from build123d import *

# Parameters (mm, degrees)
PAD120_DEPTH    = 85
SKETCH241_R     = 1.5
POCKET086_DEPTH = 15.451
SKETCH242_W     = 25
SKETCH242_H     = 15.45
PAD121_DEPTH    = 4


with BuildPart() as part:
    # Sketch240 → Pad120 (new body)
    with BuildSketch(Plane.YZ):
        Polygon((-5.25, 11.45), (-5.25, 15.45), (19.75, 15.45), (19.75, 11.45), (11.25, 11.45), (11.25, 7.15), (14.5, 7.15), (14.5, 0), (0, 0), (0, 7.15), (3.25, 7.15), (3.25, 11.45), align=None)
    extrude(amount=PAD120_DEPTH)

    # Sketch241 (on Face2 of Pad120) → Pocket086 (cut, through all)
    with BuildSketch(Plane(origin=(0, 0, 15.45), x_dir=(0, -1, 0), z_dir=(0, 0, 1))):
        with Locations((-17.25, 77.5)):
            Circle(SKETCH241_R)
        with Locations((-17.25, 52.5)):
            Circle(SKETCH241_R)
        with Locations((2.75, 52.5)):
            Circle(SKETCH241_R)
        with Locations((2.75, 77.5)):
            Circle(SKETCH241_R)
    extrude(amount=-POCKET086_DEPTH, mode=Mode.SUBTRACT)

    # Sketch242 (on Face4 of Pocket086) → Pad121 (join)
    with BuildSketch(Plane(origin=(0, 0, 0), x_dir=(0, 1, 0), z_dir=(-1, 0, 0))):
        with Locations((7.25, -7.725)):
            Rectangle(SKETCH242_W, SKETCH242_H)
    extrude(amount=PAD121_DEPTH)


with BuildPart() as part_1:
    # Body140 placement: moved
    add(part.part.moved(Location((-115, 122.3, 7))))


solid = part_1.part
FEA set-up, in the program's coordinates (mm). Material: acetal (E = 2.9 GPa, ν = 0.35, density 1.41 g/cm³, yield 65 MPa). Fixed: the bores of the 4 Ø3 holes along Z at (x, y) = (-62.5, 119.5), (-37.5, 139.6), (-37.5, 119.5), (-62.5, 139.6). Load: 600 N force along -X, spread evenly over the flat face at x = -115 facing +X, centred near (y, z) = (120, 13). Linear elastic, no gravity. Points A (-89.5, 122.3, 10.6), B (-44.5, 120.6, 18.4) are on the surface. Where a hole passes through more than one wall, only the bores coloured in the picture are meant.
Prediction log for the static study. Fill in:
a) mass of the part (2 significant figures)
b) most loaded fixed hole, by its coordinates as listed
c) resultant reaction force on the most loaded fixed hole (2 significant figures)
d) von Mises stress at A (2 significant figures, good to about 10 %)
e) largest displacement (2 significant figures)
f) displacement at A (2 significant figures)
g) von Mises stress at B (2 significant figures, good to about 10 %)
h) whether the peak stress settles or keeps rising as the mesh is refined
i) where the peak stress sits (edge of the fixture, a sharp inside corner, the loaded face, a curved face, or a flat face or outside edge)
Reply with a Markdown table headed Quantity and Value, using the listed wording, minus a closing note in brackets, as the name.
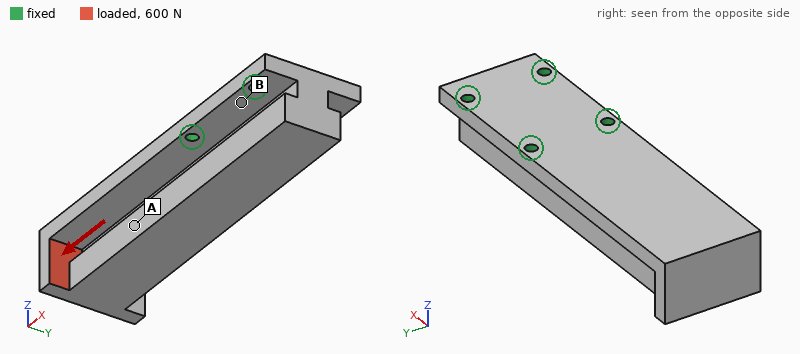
| Quantity | Value |
|---|---|
| mass of the part | 31 g |
| most loaded fixed hole, by its coordinates as listed | (-62.5, 119.5) |
| resultant reaction force on the most loaded fixed hole | 420 N |
| von Mises stress at A | 9.3 MPa |
| largest displacement | 0.85 mm |
| displacement at A | 0.24 mm |
| von Mises stress at B | 2.9 MPa |
| whether the peak stress settles or keeps rising as the mesh is refined | keeps rising |
| where the peak stress sits | edge of the fixture |
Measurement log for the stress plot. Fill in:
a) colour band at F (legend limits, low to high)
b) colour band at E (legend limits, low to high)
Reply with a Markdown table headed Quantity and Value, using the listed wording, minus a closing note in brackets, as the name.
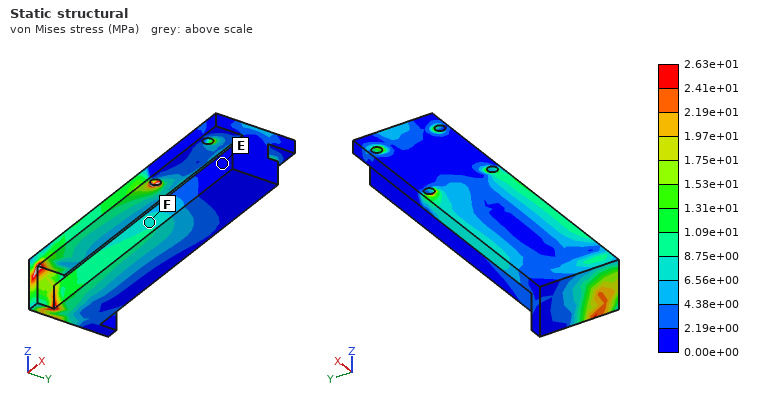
| Quantity | Value |
|---|---|
| colour band at F | 6.56e+00 to 8.75e+00 MPa |
| colour band at E | 0.00e+00 to 2.19e+00 MPa |
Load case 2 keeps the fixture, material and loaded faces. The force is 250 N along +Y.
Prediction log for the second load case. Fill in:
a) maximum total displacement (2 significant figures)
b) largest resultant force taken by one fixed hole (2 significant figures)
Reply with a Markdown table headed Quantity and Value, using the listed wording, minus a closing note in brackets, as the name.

| Quantity | Value |
|---|---|
| maximum total displacement | 1.0 mm |
| largest resultant force taken by one fixed hole | 570 N |
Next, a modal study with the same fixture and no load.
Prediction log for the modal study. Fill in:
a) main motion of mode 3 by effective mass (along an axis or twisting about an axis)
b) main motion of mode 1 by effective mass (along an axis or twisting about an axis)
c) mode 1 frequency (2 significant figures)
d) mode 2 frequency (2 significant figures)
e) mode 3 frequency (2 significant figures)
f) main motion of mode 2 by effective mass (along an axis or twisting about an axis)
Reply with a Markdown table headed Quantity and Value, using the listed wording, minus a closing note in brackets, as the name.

| Quantity | Value |
|---|---|
| main motion of mode 3 by effective mass | twisting about X |
| main motion of mode 1 by effective mass | along Z |
| mode 1 frequency | 690 Hz |
| mode 2 frequency | 1100 Hz |
| mode 3 frequency | 1900 Hz |
| main motion of mode 2 by effective mass | along Y |
